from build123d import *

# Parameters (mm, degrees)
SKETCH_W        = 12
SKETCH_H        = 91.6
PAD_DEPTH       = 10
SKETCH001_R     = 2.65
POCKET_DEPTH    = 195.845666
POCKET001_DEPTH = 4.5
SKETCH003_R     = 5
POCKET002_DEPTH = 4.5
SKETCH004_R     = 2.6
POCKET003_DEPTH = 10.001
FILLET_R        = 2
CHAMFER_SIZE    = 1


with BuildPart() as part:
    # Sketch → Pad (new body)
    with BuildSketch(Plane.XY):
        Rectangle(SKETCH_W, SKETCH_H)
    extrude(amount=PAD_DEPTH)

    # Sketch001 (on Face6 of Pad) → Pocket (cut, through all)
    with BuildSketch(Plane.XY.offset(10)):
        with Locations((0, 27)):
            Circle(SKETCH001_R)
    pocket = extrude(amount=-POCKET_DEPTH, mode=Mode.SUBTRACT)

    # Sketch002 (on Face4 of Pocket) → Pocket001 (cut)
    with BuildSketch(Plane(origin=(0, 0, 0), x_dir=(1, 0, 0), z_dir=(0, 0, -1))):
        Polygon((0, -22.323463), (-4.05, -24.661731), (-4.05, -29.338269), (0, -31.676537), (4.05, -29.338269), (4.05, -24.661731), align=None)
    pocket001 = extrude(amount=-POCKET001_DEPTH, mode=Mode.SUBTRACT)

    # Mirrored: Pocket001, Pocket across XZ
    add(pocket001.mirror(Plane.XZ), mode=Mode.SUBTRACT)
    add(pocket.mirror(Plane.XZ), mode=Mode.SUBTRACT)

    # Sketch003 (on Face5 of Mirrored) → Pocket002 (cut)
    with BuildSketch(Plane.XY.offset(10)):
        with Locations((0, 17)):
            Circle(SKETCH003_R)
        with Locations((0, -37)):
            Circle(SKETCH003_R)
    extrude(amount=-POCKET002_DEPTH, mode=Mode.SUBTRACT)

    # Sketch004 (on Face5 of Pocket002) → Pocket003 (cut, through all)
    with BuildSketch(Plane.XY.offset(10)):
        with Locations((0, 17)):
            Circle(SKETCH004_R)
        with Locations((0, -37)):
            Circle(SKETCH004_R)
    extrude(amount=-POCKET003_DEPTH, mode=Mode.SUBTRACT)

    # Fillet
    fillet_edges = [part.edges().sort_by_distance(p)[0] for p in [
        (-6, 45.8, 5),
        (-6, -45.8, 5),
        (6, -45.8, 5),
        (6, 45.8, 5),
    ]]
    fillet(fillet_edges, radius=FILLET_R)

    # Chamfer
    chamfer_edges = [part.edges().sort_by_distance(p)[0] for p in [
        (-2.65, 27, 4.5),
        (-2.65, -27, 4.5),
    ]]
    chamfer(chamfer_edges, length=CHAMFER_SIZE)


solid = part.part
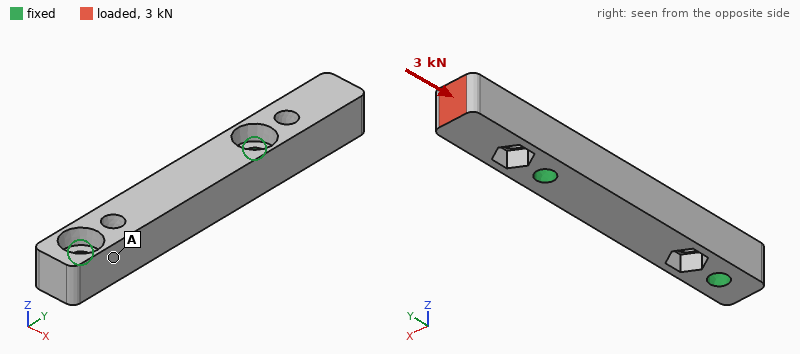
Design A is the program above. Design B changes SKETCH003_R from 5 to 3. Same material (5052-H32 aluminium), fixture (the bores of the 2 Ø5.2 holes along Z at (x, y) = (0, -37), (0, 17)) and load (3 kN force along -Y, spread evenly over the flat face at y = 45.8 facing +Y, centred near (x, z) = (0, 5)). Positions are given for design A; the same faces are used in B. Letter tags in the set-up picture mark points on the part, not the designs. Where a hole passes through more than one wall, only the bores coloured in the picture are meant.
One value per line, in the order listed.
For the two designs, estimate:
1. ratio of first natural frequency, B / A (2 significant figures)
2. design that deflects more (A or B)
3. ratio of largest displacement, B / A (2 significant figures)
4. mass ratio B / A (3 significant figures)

1.1
A
0.71
1.05
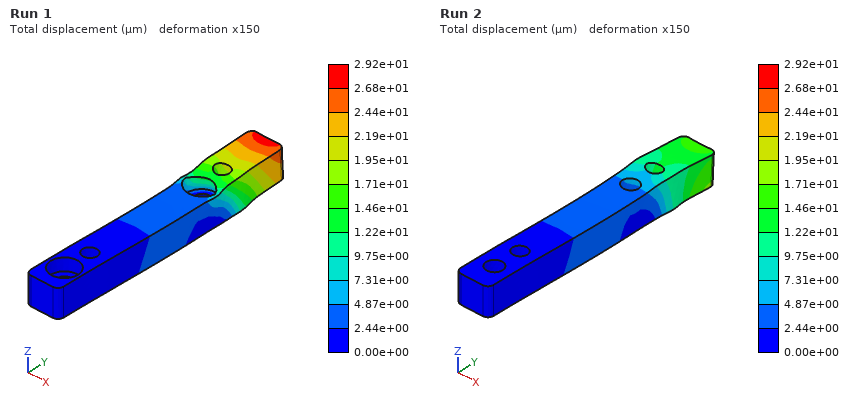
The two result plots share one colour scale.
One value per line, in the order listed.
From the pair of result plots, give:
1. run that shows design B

Run 2
